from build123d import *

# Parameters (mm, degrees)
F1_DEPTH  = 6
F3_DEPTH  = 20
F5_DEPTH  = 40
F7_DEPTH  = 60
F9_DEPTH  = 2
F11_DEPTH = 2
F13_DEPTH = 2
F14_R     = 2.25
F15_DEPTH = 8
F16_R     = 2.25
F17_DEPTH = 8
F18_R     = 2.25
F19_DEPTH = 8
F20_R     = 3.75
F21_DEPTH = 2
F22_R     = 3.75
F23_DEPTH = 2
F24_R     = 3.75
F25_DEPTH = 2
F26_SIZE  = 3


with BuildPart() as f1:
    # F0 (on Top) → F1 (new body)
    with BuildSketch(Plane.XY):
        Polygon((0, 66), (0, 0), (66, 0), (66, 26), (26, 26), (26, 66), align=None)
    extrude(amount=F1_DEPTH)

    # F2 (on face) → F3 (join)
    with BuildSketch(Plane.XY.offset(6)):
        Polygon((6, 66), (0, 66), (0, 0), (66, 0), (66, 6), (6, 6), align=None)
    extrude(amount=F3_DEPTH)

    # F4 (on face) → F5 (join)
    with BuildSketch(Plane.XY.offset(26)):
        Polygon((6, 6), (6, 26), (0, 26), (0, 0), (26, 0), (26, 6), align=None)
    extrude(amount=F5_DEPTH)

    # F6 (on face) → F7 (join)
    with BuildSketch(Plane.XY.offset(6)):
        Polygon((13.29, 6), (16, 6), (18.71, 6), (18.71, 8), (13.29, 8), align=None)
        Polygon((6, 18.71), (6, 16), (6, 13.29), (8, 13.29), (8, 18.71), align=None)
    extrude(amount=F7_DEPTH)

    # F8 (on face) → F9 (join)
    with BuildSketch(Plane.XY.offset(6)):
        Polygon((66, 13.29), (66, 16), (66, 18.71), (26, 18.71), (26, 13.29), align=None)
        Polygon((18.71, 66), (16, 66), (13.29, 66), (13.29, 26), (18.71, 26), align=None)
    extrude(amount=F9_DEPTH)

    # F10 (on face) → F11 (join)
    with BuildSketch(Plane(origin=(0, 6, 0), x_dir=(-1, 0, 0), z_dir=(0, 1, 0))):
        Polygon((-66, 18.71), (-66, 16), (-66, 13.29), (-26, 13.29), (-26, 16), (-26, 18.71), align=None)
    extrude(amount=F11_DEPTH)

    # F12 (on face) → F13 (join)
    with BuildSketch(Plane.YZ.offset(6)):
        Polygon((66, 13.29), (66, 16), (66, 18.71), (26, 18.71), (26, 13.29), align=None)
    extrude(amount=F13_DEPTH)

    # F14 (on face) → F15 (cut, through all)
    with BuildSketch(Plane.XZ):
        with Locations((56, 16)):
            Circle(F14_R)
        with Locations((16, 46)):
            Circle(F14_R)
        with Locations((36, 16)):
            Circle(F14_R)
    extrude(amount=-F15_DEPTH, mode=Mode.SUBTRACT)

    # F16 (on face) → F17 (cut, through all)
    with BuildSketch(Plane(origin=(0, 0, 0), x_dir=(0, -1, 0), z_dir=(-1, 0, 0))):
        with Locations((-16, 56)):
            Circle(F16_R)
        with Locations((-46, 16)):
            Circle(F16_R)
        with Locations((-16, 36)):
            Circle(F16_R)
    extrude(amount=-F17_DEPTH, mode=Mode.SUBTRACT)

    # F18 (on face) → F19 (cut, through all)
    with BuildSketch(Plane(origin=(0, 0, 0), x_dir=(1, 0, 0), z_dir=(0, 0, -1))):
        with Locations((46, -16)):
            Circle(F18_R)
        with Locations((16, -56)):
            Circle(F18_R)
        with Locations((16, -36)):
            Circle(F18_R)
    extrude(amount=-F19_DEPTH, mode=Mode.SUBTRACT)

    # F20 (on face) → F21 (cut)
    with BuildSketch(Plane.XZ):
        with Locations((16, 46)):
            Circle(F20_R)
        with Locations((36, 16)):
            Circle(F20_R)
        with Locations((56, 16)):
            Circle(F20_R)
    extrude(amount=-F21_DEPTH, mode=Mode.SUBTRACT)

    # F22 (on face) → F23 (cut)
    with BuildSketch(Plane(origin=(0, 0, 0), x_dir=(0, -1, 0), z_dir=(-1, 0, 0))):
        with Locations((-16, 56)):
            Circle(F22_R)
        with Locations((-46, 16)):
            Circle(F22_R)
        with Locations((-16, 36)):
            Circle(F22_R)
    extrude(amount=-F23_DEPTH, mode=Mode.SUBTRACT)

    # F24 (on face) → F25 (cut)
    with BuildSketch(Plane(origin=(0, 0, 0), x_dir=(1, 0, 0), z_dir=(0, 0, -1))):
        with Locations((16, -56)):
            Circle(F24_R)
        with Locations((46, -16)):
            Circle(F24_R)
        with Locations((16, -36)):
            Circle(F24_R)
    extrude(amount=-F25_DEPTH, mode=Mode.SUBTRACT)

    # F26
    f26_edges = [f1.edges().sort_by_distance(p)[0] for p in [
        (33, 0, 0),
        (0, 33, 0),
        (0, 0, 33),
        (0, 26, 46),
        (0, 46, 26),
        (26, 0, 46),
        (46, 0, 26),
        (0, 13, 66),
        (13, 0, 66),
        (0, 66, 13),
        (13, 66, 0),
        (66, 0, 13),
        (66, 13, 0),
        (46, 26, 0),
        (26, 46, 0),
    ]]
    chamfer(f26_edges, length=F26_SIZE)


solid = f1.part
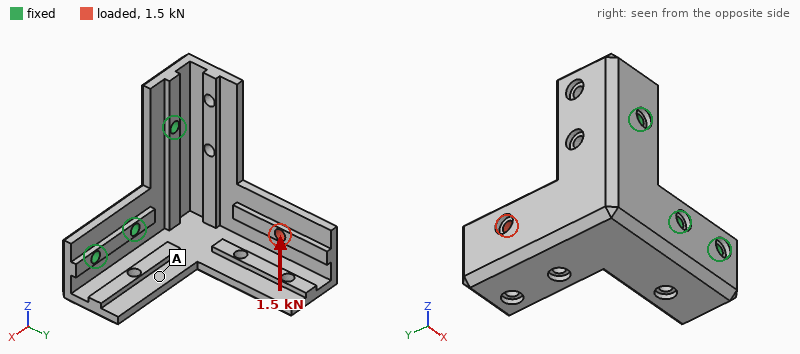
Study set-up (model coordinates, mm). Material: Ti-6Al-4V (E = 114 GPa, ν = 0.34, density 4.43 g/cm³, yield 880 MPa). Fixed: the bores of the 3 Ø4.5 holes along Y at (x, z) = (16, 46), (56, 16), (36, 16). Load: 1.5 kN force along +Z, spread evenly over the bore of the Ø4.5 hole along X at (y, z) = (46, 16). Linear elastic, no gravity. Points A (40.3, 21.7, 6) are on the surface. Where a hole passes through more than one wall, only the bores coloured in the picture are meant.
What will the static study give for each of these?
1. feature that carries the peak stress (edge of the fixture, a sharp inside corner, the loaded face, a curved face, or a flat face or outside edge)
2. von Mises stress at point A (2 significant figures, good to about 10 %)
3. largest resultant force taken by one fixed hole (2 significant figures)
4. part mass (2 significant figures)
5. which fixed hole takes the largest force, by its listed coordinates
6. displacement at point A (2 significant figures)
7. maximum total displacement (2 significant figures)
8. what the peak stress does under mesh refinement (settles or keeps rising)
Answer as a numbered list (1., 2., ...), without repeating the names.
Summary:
1. edge of the fixture
2. 26 MPa
3. 2.3 kN
4. 180 g
5. (36, 16)
6. 0.049 mm
7. 0.24 mm
8. keeps rising
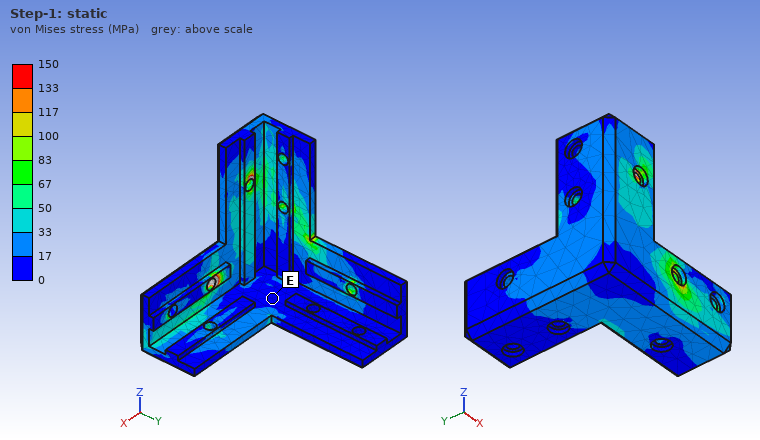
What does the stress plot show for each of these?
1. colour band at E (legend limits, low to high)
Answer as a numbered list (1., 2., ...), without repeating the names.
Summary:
1. 0 to 17 MPa
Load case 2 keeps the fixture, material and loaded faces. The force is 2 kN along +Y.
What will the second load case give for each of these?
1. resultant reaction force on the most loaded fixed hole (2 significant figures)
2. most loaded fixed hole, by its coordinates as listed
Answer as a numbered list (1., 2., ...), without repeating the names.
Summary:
1. 2.4 kN
2. (36, 16)
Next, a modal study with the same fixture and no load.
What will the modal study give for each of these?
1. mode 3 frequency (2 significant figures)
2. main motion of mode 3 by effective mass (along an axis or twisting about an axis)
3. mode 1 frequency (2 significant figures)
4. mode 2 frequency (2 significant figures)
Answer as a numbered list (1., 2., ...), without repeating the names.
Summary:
1. 5000 Hz
2. along Y
3. 1600 Hz
4. 2900 Hz
